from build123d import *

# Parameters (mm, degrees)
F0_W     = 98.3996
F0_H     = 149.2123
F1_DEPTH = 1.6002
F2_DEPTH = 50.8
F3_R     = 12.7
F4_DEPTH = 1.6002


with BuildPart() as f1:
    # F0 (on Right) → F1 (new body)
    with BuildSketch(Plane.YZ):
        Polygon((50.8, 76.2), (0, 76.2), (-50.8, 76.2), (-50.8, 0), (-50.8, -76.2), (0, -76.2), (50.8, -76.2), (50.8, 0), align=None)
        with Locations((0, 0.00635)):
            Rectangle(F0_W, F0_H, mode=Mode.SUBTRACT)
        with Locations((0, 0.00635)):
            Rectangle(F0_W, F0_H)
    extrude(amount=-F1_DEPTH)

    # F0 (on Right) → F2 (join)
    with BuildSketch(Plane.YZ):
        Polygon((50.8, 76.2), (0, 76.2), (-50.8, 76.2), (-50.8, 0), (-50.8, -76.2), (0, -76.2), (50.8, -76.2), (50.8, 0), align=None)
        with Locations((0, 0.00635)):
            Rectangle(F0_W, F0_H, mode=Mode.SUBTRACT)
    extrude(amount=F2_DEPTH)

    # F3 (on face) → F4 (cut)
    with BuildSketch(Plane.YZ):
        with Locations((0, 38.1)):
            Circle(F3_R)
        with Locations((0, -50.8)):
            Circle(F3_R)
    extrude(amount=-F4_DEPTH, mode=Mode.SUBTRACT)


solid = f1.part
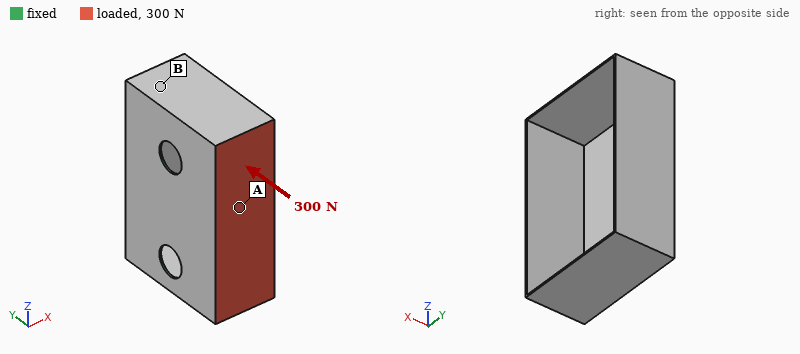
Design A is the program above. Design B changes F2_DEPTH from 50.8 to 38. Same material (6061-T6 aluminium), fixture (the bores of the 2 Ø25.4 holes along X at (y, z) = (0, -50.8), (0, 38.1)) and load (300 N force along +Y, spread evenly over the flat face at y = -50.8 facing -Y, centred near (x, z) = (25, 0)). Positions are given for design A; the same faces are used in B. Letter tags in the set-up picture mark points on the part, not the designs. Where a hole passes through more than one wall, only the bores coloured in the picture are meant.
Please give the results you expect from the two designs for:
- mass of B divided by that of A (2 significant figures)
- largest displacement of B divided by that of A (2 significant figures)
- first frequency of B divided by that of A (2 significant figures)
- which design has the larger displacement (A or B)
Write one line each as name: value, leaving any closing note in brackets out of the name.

mass of B divided by that of A: 0.84
largest displacement of B divided by that of A: 0.68
first frequency of B divided by that of A: 1.2
which design has the larger displacement: A
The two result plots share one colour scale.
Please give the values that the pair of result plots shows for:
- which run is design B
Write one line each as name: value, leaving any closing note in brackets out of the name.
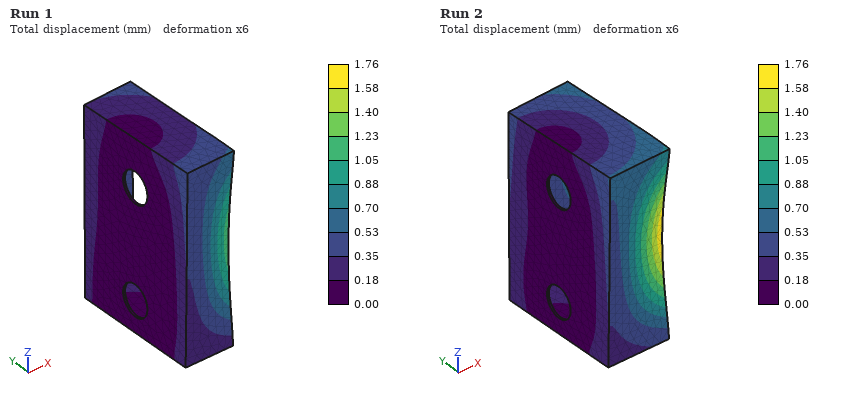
which run is design B: Run 1
